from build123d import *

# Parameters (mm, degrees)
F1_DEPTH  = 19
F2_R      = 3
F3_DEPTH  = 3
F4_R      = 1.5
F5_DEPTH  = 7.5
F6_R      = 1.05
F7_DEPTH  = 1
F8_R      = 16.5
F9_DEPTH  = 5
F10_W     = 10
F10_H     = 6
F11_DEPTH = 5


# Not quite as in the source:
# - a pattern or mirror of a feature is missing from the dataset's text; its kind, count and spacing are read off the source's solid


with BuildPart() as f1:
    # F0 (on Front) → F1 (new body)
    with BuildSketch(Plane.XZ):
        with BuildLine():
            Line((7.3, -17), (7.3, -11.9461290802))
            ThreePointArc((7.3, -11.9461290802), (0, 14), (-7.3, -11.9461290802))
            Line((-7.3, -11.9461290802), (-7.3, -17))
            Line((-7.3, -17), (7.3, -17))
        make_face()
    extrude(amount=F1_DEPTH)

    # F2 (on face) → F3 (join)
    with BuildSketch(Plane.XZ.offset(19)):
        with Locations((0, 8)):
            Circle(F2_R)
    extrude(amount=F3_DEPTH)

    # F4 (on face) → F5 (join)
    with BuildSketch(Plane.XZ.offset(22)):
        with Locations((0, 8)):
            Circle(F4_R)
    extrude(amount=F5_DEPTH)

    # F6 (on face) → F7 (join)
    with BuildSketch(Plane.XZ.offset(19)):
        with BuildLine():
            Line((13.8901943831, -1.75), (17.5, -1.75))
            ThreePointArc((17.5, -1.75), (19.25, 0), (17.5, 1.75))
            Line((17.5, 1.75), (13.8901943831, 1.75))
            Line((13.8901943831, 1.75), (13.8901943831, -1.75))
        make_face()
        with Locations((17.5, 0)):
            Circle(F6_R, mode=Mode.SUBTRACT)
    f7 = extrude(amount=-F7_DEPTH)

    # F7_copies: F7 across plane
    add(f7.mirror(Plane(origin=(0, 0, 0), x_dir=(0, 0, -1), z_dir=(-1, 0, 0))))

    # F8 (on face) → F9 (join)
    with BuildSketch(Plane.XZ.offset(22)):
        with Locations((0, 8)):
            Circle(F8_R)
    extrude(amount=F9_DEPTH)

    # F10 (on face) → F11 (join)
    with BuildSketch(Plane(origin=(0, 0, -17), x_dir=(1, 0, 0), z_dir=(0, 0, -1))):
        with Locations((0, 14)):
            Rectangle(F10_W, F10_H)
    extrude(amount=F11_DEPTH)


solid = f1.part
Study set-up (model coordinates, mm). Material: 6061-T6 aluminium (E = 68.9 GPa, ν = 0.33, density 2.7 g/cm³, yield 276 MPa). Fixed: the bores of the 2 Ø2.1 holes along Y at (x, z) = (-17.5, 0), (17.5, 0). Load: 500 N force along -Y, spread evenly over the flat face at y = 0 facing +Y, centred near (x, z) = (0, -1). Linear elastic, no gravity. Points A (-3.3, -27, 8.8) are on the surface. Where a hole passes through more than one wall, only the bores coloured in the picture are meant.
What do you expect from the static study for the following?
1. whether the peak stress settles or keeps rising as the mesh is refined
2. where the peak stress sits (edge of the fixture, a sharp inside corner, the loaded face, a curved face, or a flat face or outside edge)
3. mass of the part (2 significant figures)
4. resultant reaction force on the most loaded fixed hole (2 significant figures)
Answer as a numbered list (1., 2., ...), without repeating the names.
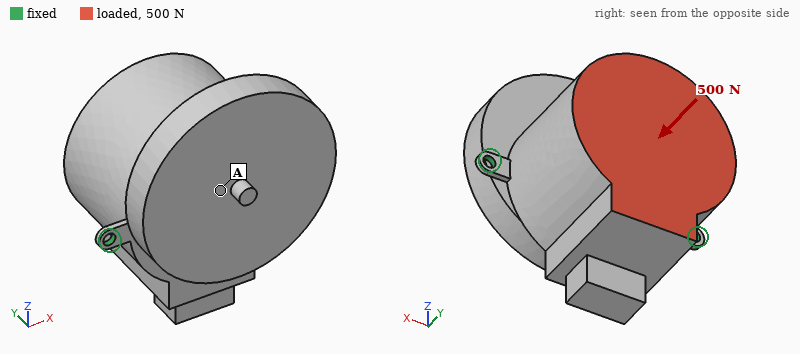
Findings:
1. keeps rising
2. edge of the fixture
3. 47 g
4. 280 N
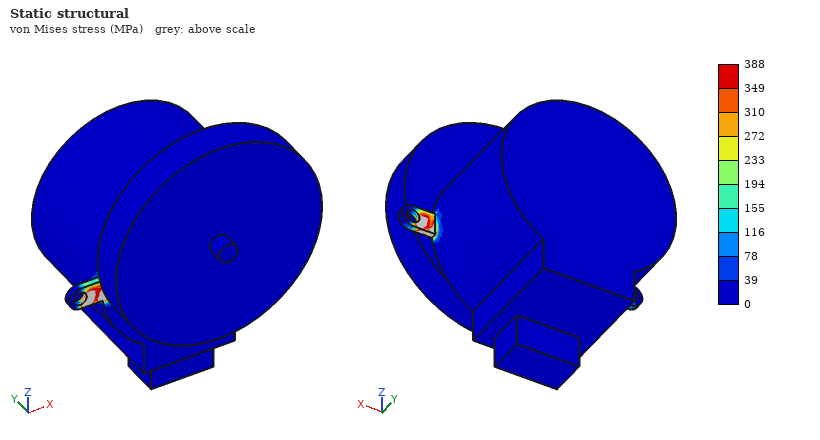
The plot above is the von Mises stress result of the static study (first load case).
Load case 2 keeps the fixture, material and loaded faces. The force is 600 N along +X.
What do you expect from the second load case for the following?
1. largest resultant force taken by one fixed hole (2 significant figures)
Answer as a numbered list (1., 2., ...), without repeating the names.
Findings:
1. 470 N
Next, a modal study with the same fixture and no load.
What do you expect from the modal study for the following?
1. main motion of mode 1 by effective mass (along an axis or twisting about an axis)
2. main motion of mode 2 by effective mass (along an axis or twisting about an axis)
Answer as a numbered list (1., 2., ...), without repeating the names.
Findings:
1. along Z
2. along Y
